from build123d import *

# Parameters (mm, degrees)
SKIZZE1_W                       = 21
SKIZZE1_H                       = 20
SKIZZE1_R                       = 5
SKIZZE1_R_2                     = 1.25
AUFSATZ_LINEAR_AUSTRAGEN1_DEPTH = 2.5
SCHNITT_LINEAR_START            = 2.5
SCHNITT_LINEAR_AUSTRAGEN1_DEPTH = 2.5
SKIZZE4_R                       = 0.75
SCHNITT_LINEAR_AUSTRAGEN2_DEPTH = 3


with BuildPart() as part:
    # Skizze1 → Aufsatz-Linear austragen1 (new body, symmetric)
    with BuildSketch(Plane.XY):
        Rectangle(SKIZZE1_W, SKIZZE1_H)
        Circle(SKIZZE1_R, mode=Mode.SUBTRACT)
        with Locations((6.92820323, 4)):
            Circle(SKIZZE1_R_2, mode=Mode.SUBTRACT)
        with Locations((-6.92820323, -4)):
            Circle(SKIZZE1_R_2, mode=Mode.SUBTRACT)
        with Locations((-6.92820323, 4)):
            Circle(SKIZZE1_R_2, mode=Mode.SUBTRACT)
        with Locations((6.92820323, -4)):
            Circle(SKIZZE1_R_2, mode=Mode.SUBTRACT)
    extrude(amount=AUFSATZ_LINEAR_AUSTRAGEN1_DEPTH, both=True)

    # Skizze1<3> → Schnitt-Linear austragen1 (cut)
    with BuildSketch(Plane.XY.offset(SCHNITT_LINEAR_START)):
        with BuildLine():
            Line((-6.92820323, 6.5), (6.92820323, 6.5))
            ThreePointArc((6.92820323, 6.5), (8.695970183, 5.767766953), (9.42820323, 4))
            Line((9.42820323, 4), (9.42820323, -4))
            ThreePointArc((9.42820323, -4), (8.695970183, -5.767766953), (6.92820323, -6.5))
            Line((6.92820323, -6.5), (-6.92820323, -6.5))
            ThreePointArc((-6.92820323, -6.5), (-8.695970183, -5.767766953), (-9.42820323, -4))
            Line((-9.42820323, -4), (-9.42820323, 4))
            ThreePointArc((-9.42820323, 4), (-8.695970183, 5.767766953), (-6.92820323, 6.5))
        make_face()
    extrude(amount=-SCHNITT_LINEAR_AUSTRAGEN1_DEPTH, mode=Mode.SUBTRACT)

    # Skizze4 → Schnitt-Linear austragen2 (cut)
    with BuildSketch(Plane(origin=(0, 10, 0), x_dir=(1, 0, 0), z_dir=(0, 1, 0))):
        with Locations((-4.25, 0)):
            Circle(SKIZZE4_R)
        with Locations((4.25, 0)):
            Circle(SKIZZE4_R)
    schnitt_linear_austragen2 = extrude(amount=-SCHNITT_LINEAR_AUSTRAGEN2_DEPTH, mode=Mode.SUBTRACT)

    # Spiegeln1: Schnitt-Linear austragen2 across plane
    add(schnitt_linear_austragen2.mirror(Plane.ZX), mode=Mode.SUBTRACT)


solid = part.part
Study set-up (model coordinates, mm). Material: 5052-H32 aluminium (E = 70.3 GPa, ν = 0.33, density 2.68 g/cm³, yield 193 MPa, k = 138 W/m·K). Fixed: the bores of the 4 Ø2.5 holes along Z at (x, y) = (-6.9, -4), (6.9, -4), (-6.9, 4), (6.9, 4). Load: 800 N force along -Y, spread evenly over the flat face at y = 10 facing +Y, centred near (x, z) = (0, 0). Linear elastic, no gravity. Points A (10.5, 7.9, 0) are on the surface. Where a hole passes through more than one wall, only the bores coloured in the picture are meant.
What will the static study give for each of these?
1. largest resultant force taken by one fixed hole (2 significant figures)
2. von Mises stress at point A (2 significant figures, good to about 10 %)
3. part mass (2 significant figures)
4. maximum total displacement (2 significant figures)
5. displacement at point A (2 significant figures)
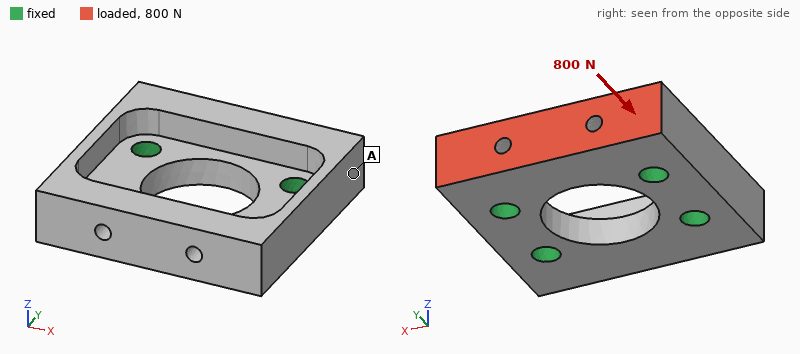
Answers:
380 N
11 MPa
3.3 g
11 µm
2.6 µm
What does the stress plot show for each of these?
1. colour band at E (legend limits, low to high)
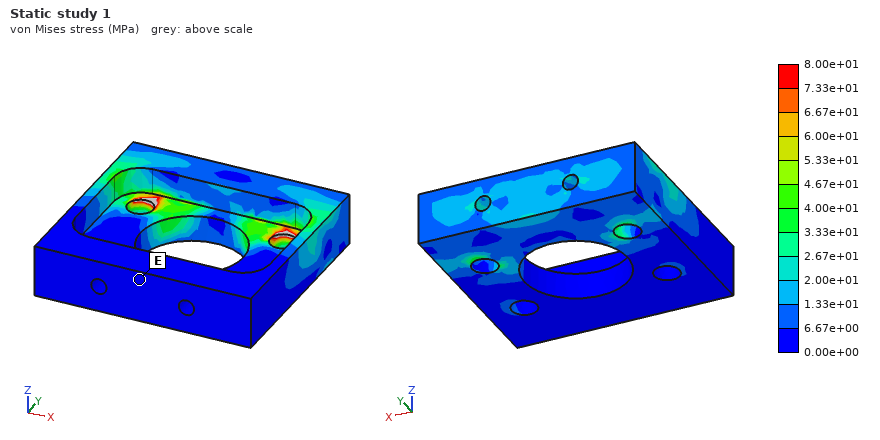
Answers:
0.00e+00 to 6.67e+00 MPa
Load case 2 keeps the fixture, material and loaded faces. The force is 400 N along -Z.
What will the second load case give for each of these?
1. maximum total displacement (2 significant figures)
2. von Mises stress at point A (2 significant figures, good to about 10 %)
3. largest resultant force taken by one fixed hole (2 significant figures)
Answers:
18 µm
21 MPa
240 N
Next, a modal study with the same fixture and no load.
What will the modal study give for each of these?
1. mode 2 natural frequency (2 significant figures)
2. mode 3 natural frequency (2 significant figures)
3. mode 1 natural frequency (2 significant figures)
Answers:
37 kHz
53 kHz
37 kHz
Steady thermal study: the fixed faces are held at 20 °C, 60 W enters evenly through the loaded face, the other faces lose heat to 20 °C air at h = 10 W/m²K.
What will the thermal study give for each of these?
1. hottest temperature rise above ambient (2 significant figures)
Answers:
52 K
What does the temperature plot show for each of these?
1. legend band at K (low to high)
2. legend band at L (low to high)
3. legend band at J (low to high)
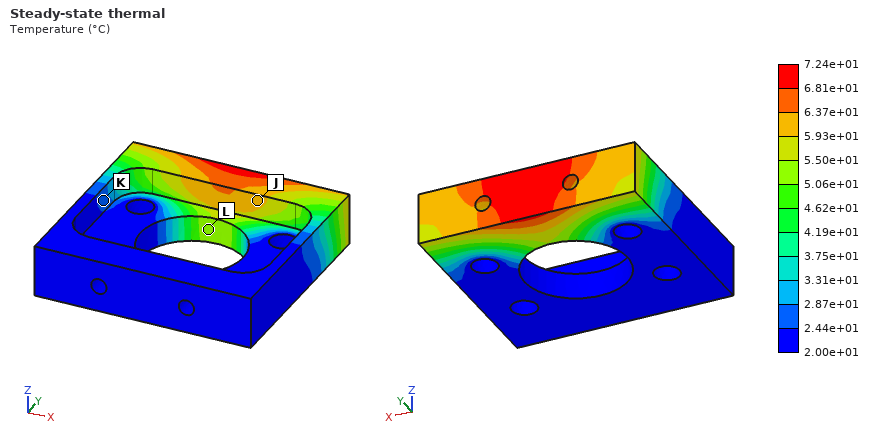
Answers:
2.44e+01 to 2.87e+01 °C
5.06e+01 to 5.50e+01 °C
5.93e+01 to 6.37e+01 °C
